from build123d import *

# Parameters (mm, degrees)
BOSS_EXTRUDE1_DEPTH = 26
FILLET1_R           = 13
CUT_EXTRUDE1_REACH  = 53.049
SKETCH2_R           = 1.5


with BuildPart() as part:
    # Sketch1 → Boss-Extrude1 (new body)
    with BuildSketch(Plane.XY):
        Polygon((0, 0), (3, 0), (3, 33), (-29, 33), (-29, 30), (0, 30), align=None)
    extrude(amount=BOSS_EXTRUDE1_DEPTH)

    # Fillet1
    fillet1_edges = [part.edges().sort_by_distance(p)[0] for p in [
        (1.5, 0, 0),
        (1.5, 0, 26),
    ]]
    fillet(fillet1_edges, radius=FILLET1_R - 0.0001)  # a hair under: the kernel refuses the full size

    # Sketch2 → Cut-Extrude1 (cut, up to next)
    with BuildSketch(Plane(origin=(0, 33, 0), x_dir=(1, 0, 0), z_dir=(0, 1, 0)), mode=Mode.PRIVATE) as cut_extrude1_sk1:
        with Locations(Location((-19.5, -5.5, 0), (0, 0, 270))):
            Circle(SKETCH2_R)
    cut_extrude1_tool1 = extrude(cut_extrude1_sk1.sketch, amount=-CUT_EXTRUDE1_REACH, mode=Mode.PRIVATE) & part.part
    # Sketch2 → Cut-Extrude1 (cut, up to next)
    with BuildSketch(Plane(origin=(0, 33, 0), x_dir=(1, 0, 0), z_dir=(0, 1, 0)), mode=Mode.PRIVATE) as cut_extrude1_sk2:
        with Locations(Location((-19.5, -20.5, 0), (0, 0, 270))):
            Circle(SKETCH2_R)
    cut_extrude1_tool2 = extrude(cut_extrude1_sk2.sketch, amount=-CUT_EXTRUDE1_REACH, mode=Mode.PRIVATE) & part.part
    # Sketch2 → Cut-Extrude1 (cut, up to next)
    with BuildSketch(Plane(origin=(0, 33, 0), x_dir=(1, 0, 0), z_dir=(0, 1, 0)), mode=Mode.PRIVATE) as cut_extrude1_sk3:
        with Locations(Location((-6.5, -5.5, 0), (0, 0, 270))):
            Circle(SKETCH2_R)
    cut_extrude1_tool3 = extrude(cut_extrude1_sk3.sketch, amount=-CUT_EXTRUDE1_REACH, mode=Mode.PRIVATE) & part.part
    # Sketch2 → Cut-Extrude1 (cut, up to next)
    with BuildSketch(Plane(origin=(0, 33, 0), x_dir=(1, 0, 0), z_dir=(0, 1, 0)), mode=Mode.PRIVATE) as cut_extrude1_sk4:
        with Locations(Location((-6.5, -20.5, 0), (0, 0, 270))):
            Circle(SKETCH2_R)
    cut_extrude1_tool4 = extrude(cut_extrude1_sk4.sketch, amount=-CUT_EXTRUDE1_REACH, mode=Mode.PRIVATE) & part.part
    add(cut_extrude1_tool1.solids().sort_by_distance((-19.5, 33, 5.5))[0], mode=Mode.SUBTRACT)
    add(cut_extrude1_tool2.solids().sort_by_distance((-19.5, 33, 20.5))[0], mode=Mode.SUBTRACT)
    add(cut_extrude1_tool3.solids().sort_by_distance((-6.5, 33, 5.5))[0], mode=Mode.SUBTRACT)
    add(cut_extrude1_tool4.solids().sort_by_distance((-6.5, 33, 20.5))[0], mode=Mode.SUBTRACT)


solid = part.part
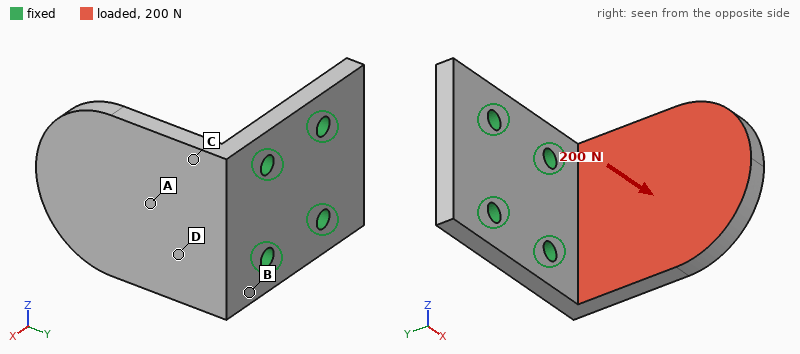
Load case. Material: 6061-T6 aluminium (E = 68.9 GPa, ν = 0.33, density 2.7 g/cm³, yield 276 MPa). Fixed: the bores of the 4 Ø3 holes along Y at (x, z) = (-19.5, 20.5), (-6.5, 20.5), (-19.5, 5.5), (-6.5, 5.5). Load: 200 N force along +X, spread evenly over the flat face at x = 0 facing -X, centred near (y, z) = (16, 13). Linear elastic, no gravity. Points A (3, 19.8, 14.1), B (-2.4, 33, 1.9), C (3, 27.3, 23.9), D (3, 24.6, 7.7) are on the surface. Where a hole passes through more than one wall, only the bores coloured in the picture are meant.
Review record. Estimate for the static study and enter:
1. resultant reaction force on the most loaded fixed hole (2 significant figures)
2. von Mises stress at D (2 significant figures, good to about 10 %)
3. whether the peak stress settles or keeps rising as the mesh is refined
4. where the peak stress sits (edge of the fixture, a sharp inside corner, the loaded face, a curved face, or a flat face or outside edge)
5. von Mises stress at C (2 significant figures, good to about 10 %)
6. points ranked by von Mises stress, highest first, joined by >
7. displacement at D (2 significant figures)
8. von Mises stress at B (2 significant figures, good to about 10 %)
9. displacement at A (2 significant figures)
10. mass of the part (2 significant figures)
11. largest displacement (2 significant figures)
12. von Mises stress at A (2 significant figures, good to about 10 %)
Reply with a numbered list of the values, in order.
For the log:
1. 94 N
2. 41 MPa
3. keeps rising
4. edge of the fixture
5. 55 MPa
6. B > C > D > A
7. 0.059 mm
8. 70 MPa
9. 0.10 mm
10. 12 g
11. 0.32 mm
12. 24 MPa
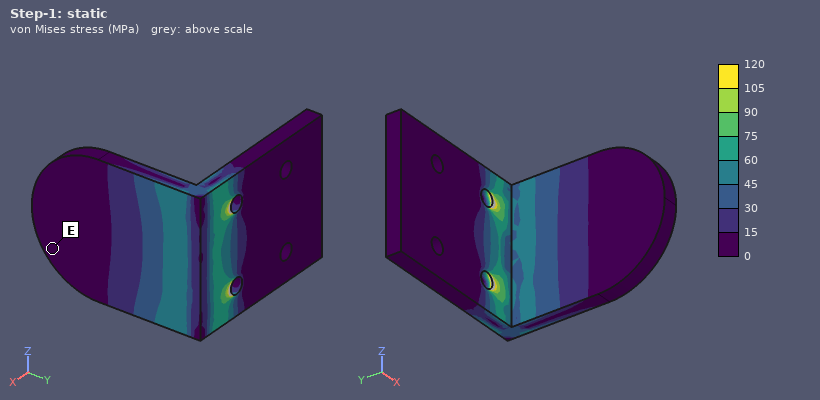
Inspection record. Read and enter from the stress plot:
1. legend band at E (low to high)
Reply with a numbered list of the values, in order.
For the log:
1. 0 to 15 MPa
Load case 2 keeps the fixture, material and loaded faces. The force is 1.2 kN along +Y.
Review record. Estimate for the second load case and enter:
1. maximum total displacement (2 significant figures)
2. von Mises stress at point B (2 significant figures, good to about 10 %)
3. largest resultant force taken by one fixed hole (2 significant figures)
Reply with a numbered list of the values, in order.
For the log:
1. 69 µm
2. 65 MPa
3. 660 N
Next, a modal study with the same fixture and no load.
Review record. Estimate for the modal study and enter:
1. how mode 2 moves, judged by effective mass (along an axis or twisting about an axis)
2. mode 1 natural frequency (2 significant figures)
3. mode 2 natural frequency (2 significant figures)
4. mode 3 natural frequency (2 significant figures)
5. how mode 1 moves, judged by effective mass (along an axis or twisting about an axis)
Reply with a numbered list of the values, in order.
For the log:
1. along Z
2. 2100 Hz
3. 5500 Hz
4. 8500 Hz
5. along X
